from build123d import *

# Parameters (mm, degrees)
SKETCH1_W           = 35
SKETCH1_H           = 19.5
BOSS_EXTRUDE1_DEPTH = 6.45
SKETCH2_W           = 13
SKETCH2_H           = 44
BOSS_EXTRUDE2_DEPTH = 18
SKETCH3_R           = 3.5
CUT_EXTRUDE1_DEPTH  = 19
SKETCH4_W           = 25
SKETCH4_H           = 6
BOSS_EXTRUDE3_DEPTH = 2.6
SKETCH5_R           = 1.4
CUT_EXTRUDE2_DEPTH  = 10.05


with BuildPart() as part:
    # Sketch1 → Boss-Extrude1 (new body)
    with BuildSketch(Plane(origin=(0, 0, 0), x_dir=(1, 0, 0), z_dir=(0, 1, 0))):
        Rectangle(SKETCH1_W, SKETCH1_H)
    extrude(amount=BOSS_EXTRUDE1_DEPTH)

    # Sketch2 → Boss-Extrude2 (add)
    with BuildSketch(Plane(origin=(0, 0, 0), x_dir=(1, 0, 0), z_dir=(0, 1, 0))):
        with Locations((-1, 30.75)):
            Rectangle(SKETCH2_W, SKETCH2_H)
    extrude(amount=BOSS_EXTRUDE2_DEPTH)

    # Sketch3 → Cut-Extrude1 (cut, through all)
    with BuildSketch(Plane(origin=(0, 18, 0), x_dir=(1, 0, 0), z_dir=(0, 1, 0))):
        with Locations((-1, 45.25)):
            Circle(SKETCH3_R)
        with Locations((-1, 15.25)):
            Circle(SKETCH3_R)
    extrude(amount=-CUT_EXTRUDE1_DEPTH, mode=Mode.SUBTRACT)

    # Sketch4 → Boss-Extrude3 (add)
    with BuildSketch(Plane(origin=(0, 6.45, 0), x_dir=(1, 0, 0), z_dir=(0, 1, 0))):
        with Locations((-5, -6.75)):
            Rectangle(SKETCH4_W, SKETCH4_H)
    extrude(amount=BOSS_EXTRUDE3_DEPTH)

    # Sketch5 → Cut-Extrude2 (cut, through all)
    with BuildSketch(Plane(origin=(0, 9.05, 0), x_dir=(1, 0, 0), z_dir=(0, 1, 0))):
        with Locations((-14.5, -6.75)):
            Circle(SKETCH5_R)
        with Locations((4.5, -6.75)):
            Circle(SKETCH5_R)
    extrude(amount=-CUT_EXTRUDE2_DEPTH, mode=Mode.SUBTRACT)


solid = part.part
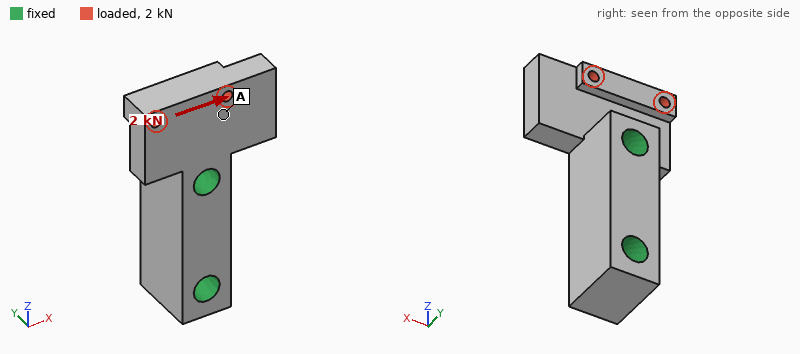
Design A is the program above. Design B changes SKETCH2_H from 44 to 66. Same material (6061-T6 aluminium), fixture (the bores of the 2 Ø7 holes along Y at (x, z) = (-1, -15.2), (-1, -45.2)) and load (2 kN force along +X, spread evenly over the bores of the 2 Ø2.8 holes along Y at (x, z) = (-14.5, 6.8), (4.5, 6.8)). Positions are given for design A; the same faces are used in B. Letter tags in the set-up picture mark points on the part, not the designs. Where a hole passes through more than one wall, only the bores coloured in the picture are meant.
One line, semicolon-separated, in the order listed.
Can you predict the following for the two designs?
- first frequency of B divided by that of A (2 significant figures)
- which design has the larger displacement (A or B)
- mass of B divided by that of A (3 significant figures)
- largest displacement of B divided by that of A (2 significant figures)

1.5; A; 1.31; 0.56
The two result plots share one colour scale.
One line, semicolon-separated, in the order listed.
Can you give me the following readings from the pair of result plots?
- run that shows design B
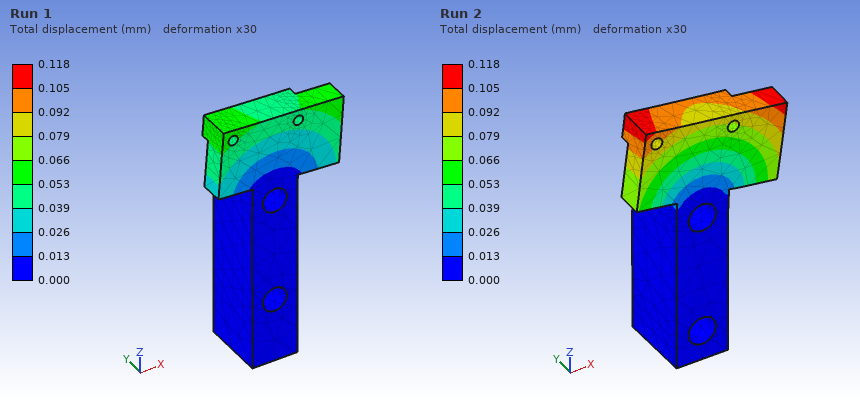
Run 1
